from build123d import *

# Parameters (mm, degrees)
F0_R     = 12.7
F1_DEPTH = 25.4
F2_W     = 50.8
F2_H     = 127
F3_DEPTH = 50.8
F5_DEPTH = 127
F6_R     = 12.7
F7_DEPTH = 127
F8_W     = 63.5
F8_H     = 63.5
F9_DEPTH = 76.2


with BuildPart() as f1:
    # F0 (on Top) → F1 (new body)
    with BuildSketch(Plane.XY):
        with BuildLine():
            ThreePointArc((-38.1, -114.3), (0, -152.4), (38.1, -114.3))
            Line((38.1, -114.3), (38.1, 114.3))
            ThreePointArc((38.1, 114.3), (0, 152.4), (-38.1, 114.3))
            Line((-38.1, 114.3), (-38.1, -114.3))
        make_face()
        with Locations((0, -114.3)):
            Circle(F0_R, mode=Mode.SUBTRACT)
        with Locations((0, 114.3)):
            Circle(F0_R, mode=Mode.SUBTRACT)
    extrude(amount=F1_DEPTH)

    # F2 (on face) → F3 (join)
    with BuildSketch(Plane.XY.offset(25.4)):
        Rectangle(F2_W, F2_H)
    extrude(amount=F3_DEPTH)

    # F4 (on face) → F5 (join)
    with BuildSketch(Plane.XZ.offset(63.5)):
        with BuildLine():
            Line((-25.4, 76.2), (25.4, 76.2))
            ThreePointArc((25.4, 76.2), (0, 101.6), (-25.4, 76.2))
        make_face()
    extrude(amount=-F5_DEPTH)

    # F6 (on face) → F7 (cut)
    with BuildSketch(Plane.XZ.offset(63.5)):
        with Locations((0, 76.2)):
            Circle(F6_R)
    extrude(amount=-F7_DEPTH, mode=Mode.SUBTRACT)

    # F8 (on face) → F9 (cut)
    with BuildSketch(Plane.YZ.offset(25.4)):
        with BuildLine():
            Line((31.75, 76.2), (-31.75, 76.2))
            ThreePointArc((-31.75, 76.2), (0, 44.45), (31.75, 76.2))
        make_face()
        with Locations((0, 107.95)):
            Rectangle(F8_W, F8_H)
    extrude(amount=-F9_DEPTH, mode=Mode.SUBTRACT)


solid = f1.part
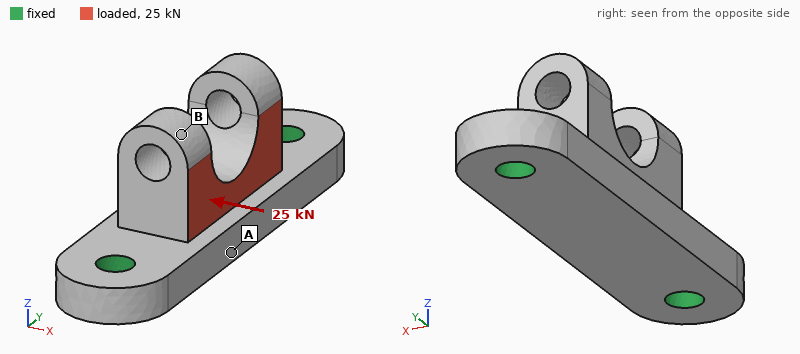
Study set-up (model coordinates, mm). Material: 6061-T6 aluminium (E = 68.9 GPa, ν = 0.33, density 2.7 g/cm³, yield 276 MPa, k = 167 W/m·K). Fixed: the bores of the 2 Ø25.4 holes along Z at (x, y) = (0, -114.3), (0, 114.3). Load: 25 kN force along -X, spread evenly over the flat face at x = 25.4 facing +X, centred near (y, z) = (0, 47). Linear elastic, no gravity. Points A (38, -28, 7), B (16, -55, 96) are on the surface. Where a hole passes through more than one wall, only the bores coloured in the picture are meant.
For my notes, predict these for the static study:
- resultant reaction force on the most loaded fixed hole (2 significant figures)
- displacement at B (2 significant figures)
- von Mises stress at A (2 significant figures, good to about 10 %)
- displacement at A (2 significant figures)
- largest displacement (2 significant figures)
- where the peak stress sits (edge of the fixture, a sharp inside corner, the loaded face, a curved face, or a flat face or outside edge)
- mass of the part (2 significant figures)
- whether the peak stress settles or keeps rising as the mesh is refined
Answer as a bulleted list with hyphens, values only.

- 13 kN
- 0.24 mm
- 19 MPa
- 0.093 mm
- 0.26 mm
- edge of the fixture
- 2.2 kg
- keeps rising
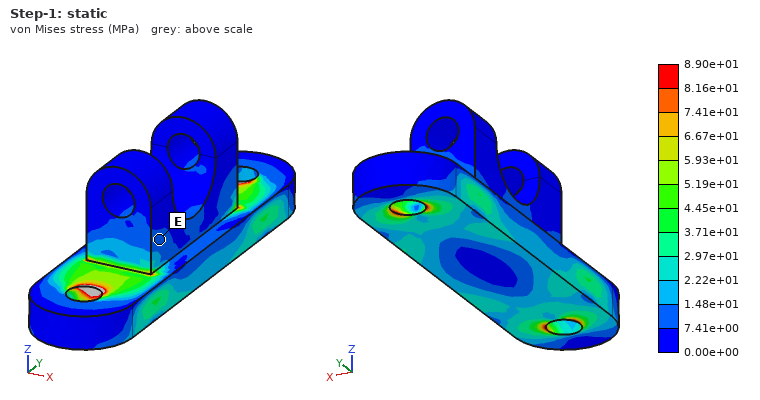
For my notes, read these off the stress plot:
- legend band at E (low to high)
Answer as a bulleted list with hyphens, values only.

- 7.41e+00 to 1.48e+01 MPa
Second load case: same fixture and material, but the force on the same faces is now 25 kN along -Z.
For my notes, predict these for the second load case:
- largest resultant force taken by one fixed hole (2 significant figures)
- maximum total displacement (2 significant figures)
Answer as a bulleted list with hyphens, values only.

- 14 kN
- 0.19 mm
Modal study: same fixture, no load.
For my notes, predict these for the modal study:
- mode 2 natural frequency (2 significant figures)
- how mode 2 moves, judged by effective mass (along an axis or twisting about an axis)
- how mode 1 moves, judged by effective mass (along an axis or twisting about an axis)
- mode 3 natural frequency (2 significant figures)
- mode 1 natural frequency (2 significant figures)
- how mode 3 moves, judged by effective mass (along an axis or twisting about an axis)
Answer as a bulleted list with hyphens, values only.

- 2500 Hz
- along Z
- along X
- 4000 Hz
- 1900 Hz
- along X
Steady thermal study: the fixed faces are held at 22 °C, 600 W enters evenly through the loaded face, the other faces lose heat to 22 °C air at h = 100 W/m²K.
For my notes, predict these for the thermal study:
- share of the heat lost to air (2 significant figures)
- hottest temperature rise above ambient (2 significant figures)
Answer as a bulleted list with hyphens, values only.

- 38 %
- 62 K
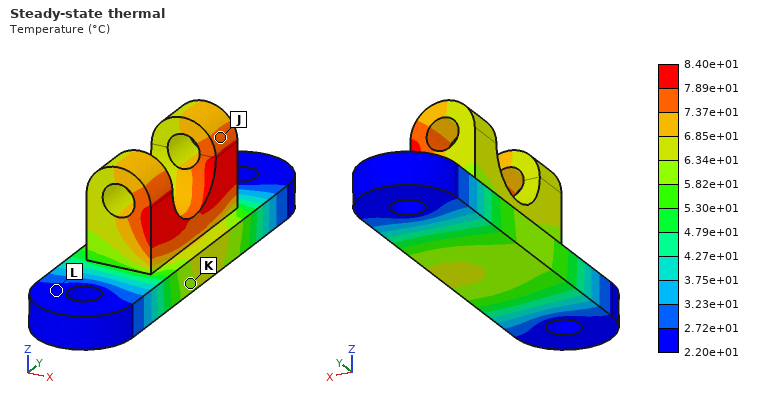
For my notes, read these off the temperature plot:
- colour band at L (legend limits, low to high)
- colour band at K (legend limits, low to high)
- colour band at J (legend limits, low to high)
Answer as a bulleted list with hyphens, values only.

- 2.20e+01 to 2.72e+01 °C
- 5.82e+01 to 6.34e+01 °C
- 7.37e+01 to 7.89e+01 °C
